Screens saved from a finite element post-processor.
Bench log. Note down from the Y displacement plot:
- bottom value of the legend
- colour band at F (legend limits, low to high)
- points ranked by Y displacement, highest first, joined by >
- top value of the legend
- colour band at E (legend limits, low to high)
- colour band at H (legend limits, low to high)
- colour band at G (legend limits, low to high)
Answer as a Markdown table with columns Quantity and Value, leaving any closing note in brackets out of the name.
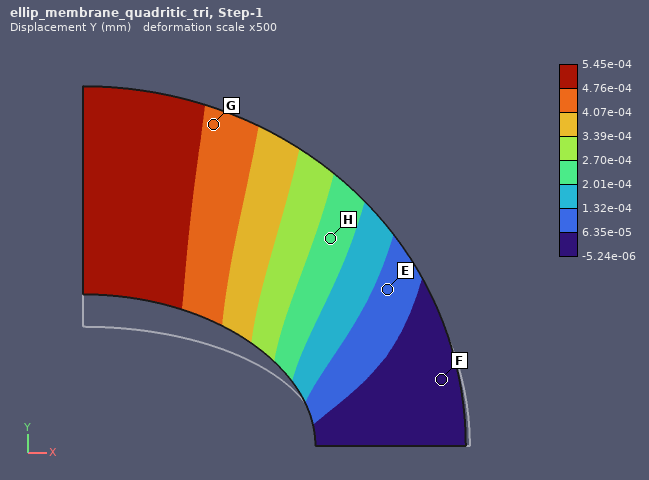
| Quantity | Value |
|---|---|
| bottom value of the legend | -5.24e-06 mm |
| colour band at F | -5.24e-06 to 6.35e-05 mm |
| points ranked by Y displacement, highest first, joined by > | G > H > E > F |
| top value of the legend | 5.45e-04 mm |
| colour band at E | 6.35e-05 to 1.32e-04 mm |
| colour band at H | 2.01e-04 to 2.70e-04 mm |
| colour band at G | 4.07e-04 to 4.76e-04 mm |
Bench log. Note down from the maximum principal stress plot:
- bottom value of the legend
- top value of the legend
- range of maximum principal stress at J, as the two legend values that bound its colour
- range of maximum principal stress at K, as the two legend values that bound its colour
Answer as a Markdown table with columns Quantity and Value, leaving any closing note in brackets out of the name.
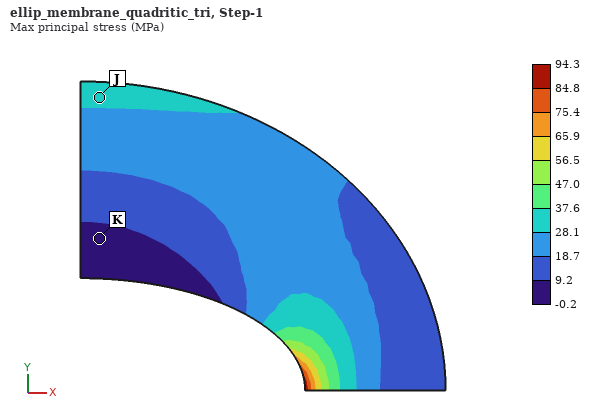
| Quantity | Value |
|---|---|
| bottom value of the legend | -0.2 MPa |
| top value of the legend | 94.3 MPa |
| range of maximum principal stress at J, as the two legend values that bound its colour | 28.1 to 37.6 MPa |
| range of maximum principal stress at K, as the two legend values that bound its colour | -0.2 to 9.2 MPa |
